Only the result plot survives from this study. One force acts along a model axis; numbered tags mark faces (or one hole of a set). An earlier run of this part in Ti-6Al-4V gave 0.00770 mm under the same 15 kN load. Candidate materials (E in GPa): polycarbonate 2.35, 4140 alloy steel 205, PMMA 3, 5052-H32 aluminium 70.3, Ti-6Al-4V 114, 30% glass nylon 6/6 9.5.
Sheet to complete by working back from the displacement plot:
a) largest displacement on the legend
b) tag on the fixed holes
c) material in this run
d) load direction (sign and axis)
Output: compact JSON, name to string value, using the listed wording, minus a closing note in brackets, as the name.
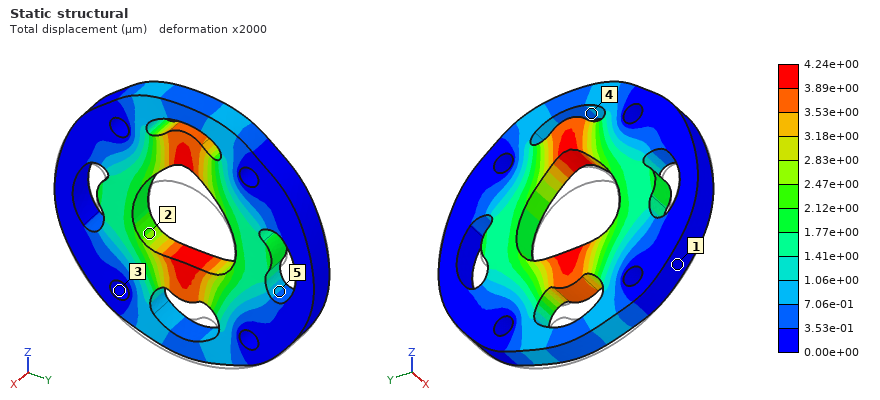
{"largest displacement on the legend": "4.24e+00 µm", "tag on the fixed holes": "3", "material in this run": "4140 alloy steel", "load direction": "+Z"}
